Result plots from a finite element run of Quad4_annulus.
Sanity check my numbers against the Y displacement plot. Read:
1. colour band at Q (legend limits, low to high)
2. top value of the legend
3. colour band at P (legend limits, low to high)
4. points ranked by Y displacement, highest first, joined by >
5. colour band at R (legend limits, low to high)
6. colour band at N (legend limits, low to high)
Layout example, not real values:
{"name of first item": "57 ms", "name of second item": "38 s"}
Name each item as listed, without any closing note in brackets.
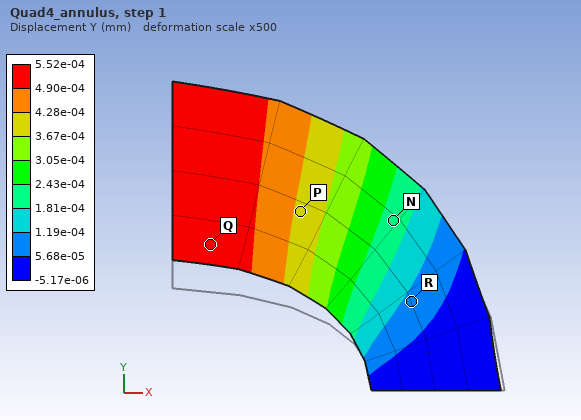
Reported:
{"colour band at Q": "4.90e-04 to 5.52e-04 mm", "top value of the legend": "5.52e-04 mm", "colour band at P": "3.67e-04 to 4.28e-04 mm", "points ranked by Y displacement, highest first, joined by >": "Q > P > N > R", "colour band at R": "5.68e-05 to 1.19e-04 mm", "colour band at N": "1.81e-04 to 2.43e-04 mm"}
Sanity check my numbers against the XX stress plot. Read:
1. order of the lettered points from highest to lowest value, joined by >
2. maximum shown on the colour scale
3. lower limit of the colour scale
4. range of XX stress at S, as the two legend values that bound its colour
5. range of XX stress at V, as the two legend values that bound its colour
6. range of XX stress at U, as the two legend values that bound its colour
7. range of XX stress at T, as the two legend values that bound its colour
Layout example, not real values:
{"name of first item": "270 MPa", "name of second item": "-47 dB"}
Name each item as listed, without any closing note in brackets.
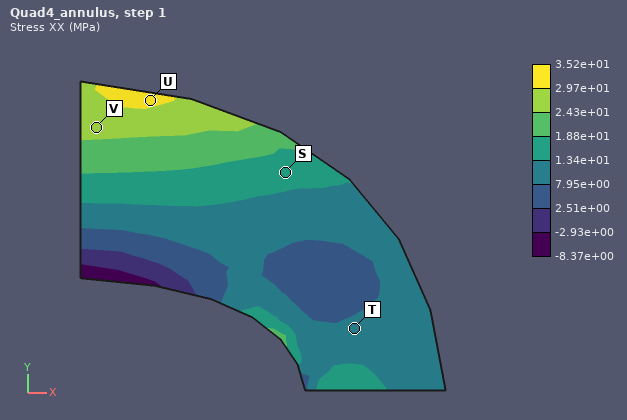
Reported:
{"order of the lettered points from highest to lowest value, joined by >": "U > V > S > T", "maximum shown on the colour scale": "3.52e+01 MPa", "lower limit of the colour scale": "-8.37e+00 MPa", "range of XX stress at S, as the two legend values that bound its colour": "1.34e+01 to 1.88e+01 MPa", "range of XX stress at V, as the two legend values that bound its colour": "2.43e+01 to 2.97e+01 MPa", "range of XX stress at U, as the two legend values that bound its colour": "2.97e+01 to 3.52e+01 MPa", "range of XX stress at T, as the two legend values that bound its colour": "7.95e+00 to 1.34e+01 MPa"}
